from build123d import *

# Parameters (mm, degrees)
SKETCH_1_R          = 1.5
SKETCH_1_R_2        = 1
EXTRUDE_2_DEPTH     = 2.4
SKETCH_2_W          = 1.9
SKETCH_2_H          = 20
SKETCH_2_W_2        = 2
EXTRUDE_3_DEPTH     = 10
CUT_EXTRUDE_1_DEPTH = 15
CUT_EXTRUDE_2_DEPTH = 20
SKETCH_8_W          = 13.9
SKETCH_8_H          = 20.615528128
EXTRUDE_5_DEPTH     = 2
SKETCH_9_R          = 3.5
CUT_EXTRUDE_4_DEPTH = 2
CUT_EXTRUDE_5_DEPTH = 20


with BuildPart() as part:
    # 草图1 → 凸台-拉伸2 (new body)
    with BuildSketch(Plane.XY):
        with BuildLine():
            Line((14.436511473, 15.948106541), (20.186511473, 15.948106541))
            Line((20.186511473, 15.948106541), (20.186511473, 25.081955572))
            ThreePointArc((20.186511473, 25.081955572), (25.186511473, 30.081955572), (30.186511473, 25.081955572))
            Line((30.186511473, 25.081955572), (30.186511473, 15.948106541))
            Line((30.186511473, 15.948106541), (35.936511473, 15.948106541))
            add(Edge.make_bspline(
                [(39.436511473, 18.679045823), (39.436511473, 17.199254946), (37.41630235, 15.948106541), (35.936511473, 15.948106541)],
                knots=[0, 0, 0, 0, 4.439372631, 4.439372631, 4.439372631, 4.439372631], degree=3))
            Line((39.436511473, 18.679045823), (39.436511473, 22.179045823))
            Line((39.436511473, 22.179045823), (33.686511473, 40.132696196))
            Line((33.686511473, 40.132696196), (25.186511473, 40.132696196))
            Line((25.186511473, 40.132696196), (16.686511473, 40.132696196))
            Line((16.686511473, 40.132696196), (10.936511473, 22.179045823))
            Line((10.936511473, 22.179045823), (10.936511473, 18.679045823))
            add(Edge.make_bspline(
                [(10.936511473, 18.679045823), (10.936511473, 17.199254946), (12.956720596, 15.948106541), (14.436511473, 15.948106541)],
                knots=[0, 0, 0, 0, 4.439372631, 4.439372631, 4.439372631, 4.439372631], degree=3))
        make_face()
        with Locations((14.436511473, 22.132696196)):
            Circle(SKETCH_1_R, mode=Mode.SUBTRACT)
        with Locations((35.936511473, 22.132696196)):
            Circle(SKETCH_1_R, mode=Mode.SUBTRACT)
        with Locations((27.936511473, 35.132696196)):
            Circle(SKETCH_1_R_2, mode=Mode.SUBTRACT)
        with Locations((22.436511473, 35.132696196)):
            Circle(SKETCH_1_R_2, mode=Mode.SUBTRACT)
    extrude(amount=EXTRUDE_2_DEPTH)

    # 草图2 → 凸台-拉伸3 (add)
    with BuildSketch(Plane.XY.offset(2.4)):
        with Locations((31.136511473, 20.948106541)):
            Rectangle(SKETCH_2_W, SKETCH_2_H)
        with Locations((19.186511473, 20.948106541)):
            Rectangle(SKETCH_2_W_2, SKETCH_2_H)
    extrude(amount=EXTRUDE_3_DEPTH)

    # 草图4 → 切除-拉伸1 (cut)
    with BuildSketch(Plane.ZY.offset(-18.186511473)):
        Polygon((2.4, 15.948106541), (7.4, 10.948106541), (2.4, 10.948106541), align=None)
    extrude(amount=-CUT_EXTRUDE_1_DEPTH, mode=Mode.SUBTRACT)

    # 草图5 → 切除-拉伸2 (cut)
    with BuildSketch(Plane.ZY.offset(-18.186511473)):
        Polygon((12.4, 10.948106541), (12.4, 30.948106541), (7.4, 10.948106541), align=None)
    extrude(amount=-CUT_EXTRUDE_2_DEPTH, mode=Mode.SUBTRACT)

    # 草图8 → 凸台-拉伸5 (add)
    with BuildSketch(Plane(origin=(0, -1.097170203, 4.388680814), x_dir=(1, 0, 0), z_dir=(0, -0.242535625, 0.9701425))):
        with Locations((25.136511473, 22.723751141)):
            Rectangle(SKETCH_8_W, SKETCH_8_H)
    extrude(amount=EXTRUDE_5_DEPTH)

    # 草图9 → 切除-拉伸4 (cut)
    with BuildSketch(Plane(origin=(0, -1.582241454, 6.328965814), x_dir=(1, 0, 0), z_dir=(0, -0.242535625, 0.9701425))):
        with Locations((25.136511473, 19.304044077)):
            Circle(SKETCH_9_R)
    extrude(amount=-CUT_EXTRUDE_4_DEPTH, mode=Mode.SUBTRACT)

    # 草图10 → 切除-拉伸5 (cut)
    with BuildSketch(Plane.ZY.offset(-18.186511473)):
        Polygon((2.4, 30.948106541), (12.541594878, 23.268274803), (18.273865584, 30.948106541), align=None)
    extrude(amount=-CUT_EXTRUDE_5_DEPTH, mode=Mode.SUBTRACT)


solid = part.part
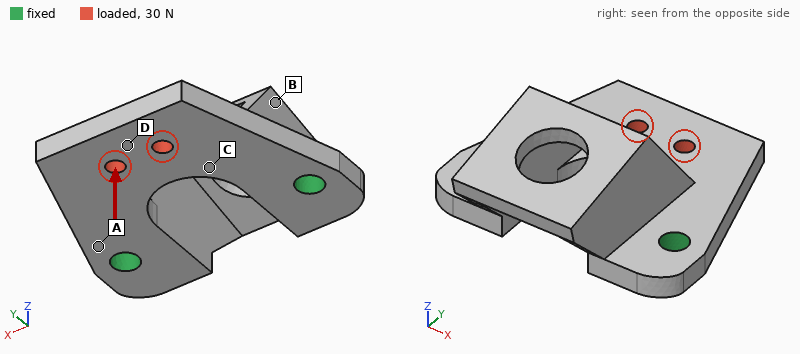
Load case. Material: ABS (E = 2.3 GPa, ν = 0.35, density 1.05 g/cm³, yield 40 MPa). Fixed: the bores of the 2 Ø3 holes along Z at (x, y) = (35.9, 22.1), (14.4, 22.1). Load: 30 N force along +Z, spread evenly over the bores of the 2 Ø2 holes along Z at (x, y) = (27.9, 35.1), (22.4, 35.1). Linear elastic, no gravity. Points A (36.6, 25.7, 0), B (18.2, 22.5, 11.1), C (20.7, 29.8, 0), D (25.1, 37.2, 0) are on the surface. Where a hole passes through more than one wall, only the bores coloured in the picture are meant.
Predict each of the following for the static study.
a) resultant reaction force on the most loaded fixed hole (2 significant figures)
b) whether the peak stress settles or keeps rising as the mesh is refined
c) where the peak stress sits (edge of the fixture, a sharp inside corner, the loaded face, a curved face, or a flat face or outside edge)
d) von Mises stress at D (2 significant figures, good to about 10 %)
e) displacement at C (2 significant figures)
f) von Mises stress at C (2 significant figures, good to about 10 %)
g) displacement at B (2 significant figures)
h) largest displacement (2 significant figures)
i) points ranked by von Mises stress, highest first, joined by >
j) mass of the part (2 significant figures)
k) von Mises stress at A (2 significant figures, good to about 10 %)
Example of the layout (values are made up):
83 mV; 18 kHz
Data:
15 N; keeps rising; edge of the fixture; 4.9 MPa; 0.15 mm; 8.0 MPa; 0.14 mm; 0.49 mm; A > C > D > B; 1.8 g; 11 MPa
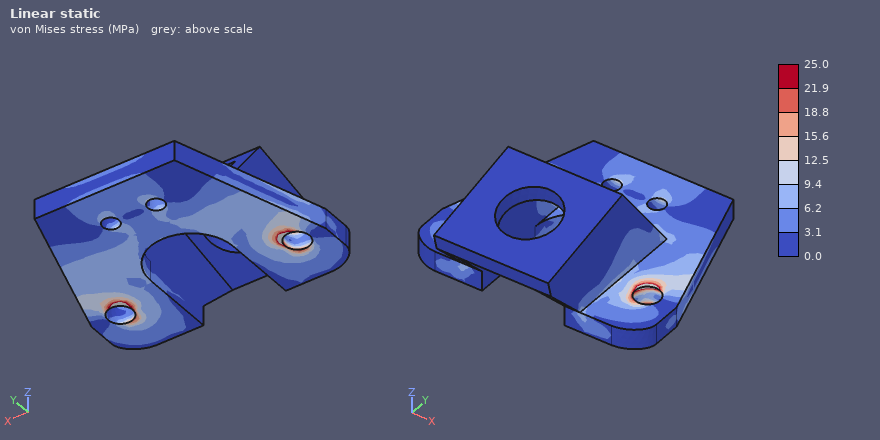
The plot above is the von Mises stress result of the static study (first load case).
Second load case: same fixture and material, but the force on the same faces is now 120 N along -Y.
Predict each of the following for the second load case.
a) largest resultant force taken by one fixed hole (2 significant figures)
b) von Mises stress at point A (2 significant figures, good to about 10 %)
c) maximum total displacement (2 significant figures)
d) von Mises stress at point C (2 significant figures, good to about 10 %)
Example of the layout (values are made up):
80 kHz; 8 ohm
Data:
67 N; 3.3 MPa; 40 µm; 4.7 MPa
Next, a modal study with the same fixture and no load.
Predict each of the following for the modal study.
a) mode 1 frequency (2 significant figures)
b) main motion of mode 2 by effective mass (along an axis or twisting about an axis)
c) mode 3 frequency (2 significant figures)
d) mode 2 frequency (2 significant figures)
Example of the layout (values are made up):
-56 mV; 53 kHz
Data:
2000 Hz; along X; 4800 Hz; 4100 Hz
